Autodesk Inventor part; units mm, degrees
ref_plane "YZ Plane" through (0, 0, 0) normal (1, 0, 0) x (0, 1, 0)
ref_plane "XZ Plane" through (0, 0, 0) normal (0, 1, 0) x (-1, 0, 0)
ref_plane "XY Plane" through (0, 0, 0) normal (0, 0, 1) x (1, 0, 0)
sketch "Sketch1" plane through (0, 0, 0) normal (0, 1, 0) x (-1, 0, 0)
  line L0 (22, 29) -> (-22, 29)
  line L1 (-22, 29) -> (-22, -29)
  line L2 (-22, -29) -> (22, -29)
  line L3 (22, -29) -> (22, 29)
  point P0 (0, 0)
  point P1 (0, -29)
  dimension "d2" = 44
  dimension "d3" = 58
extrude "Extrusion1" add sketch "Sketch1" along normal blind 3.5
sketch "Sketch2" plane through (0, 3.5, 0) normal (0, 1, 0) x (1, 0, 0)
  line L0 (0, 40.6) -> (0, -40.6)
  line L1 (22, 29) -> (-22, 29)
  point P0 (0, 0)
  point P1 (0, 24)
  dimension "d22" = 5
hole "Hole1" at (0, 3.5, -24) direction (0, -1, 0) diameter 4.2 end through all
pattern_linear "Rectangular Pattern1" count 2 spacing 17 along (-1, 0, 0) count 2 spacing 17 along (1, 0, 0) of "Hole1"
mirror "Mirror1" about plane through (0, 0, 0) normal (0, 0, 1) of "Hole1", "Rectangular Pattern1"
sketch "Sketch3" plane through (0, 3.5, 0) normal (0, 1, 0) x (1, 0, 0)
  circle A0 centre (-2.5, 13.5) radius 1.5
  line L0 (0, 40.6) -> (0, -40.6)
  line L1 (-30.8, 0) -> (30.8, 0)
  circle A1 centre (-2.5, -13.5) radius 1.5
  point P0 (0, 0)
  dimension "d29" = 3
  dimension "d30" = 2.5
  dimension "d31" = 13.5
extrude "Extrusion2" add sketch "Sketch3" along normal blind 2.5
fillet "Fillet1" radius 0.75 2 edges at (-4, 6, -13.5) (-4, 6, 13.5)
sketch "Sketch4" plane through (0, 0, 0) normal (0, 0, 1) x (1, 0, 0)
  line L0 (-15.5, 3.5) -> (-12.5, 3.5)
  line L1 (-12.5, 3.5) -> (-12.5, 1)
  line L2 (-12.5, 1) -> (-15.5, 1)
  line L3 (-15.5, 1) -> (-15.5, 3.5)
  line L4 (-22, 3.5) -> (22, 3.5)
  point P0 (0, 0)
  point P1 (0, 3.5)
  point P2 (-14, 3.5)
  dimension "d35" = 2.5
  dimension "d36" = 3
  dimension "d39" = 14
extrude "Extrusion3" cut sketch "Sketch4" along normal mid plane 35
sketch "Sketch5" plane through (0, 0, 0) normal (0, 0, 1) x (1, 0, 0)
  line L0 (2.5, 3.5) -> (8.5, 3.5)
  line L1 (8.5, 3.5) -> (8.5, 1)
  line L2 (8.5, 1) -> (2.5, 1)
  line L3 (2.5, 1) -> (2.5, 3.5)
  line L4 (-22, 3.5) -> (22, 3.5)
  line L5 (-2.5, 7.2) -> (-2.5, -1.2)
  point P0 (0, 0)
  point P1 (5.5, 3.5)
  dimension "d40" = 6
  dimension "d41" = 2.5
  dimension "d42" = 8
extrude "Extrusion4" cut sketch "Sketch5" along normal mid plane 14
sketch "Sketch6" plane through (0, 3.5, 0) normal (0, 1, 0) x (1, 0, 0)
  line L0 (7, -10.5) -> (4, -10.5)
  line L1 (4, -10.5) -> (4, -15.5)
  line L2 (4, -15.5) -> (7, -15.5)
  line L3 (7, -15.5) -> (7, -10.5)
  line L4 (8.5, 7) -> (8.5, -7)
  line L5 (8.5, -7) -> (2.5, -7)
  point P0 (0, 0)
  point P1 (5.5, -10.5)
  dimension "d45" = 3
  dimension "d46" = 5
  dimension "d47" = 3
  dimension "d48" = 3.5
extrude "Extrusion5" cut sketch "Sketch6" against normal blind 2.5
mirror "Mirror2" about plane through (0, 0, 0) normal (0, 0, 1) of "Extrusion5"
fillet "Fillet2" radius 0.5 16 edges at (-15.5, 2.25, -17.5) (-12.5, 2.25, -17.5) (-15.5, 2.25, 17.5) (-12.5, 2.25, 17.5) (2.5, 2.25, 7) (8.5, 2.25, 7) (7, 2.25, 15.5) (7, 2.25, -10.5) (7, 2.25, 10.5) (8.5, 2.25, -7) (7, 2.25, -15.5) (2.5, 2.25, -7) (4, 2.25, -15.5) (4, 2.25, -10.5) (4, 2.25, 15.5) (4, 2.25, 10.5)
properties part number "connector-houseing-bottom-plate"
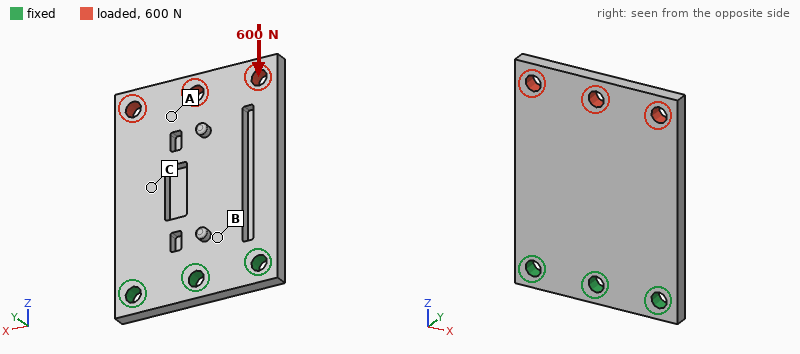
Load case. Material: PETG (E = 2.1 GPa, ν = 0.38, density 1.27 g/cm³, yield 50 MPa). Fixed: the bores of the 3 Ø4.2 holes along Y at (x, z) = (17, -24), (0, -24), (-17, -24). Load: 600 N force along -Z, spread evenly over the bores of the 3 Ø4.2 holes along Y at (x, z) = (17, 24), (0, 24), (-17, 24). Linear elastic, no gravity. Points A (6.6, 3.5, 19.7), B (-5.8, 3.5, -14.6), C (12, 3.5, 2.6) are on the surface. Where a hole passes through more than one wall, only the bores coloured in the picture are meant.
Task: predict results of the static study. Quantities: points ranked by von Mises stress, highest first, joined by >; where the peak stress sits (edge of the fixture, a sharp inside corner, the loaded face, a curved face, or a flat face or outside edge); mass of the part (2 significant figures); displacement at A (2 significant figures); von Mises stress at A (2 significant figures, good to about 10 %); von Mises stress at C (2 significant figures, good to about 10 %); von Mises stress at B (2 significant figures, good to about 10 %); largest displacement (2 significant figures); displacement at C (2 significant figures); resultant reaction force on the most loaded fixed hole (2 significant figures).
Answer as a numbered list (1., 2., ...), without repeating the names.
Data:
1. C > B > A
2. a curved face
3. 10 g
4. 0.14 mm
5. 2.2 MPa
6. 5.4 MPa
7. 3.9 MPa
8. 0.21 mm
9. 0.069 mm
10. 210 N
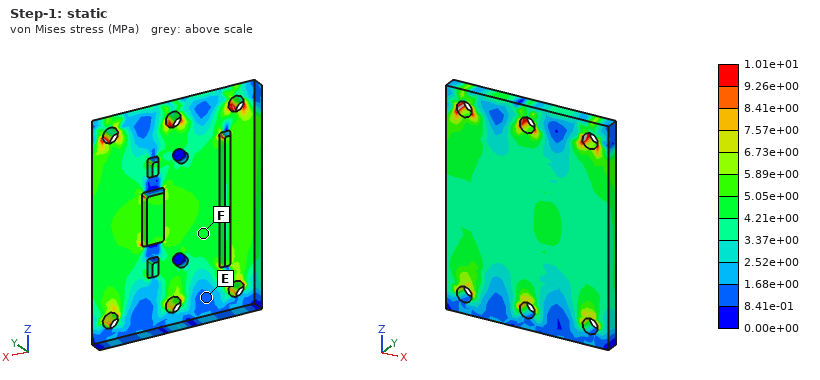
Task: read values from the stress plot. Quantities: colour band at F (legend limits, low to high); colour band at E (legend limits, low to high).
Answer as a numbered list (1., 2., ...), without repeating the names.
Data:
1. 4.21e+00 to 5.05e+00 MPa
2. 8.41e-01 to 1.68e+00 MPa
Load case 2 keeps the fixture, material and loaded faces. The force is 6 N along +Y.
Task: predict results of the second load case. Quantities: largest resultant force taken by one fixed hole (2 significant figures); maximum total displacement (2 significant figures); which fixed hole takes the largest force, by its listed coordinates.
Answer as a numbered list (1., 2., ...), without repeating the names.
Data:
1. 4.9 N
2. 0.76 mm
3. (0, -24)
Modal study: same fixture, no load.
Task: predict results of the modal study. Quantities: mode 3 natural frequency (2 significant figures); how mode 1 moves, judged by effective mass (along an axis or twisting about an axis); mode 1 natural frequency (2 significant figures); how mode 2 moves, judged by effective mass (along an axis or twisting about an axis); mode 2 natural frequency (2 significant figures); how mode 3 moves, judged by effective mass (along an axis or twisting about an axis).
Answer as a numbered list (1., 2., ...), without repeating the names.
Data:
1. 1700 Hz
2. along Y
3. 280 Hz
4. twisting about Z
5. 700 Hz
6. along Y
